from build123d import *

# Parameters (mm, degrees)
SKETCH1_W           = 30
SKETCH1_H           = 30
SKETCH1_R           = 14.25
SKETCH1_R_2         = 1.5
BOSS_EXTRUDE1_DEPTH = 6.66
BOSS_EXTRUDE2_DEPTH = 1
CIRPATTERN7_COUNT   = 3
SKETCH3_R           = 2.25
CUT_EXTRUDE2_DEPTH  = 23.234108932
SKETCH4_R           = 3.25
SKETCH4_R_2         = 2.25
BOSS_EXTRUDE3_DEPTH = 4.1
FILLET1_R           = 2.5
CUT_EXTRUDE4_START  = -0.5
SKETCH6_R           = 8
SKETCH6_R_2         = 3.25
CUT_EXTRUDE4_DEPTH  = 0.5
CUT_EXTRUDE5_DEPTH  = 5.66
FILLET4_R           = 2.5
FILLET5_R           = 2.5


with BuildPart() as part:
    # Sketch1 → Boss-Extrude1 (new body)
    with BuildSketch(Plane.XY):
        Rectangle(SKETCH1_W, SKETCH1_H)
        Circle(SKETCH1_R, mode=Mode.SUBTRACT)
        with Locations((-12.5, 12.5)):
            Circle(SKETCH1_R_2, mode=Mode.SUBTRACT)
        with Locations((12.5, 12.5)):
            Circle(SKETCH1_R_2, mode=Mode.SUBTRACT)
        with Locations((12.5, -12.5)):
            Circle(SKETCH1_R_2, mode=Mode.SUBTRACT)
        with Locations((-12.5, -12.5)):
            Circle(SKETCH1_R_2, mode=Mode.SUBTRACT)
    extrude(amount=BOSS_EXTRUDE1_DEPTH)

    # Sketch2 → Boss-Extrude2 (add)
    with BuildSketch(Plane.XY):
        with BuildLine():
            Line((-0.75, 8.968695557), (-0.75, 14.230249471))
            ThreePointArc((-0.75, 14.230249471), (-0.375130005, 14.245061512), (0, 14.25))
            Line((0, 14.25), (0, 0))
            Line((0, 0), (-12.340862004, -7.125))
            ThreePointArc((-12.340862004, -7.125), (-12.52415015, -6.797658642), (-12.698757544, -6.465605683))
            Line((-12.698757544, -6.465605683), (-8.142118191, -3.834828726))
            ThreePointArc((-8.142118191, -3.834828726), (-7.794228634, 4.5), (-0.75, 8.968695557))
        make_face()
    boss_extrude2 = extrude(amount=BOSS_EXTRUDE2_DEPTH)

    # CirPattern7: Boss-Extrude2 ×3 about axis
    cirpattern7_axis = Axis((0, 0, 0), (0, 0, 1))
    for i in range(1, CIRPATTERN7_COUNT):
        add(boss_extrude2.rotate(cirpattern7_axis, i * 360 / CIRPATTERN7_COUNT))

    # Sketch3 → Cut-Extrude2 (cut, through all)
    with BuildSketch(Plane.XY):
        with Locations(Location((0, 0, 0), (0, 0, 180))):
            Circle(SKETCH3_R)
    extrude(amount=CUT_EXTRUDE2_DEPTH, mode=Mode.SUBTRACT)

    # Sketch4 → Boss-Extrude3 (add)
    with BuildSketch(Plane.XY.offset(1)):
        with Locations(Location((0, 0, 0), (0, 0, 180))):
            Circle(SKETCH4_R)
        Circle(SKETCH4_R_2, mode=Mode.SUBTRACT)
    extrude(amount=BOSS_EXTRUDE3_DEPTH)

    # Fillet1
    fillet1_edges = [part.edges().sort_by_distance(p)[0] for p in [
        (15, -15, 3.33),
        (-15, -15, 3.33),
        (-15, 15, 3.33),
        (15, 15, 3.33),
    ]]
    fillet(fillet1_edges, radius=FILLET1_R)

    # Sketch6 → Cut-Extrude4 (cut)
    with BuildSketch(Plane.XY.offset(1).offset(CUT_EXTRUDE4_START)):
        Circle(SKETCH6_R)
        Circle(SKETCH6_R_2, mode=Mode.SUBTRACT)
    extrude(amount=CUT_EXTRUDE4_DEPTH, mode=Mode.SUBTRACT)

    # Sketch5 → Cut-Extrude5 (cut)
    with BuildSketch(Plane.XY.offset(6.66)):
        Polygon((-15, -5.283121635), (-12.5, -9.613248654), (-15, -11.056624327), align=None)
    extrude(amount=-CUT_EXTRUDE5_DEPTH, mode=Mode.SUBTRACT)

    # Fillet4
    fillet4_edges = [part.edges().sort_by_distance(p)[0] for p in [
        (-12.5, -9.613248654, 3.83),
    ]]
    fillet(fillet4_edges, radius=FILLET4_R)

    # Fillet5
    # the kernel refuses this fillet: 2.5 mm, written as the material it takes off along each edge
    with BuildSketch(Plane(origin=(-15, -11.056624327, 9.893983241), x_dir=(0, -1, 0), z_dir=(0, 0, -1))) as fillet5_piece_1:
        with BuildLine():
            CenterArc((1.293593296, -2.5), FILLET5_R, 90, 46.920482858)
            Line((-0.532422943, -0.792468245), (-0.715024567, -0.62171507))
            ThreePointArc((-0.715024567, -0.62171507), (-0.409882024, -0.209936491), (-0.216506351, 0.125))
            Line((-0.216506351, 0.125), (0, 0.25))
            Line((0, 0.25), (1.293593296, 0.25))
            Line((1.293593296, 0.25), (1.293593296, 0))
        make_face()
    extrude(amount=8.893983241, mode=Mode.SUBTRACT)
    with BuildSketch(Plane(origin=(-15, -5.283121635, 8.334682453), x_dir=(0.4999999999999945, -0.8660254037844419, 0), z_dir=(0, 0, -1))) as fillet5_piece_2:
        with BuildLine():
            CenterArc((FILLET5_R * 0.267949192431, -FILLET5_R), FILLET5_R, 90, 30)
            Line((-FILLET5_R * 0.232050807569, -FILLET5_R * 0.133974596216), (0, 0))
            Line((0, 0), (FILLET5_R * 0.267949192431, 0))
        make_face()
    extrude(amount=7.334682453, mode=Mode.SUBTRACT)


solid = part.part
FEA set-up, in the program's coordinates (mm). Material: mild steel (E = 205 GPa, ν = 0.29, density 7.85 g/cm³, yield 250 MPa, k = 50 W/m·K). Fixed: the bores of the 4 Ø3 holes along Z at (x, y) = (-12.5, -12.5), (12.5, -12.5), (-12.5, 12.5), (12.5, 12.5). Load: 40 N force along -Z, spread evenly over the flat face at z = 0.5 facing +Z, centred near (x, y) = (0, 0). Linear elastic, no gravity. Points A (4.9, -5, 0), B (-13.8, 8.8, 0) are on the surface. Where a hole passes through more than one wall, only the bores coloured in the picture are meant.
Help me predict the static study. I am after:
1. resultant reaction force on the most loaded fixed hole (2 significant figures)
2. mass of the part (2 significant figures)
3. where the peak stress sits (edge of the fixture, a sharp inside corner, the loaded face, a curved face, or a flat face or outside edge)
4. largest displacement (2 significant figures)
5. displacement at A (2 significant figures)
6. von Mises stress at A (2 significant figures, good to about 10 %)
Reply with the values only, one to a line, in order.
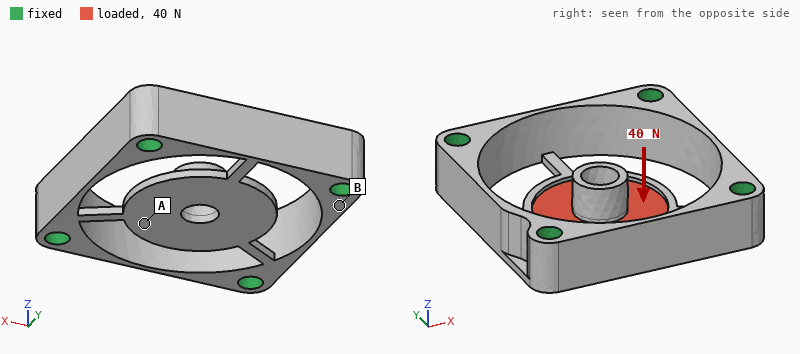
29 N
14 g
a flat face or outside edge
46 µm
35 µm
49 MPa
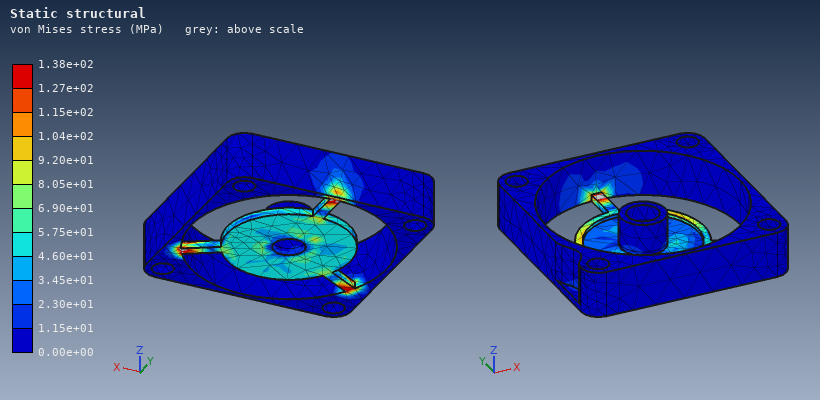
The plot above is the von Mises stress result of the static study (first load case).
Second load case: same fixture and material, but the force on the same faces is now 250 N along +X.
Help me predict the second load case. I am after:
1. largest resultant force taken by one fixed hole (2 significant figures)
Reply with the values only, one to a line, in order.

130 N
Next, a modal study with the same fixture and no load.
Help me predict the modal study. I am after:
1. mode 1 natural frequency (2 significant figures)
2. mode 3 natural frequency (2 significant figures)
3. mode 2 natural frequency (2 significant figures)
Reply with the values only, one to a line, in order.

3700 Hz
6000 Hz
5800 Hz
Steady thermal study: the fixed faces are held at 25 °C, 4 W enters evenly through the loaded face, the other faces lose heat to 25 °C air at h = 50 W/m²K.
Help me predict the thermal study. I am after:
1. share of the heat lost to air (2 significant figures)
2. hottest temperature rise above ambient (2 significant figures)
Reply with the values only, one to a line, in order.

53 %
73 K
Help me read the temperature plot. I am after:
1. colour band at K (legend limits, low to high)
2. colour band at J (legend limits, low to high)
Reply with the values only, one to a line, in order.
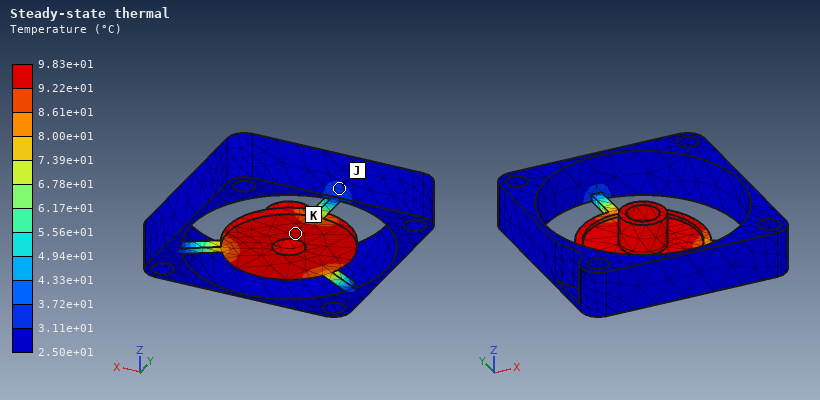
9.22e+01 to 9.83e+01 °C
3.11e+01 to 3.72e+01 °C
